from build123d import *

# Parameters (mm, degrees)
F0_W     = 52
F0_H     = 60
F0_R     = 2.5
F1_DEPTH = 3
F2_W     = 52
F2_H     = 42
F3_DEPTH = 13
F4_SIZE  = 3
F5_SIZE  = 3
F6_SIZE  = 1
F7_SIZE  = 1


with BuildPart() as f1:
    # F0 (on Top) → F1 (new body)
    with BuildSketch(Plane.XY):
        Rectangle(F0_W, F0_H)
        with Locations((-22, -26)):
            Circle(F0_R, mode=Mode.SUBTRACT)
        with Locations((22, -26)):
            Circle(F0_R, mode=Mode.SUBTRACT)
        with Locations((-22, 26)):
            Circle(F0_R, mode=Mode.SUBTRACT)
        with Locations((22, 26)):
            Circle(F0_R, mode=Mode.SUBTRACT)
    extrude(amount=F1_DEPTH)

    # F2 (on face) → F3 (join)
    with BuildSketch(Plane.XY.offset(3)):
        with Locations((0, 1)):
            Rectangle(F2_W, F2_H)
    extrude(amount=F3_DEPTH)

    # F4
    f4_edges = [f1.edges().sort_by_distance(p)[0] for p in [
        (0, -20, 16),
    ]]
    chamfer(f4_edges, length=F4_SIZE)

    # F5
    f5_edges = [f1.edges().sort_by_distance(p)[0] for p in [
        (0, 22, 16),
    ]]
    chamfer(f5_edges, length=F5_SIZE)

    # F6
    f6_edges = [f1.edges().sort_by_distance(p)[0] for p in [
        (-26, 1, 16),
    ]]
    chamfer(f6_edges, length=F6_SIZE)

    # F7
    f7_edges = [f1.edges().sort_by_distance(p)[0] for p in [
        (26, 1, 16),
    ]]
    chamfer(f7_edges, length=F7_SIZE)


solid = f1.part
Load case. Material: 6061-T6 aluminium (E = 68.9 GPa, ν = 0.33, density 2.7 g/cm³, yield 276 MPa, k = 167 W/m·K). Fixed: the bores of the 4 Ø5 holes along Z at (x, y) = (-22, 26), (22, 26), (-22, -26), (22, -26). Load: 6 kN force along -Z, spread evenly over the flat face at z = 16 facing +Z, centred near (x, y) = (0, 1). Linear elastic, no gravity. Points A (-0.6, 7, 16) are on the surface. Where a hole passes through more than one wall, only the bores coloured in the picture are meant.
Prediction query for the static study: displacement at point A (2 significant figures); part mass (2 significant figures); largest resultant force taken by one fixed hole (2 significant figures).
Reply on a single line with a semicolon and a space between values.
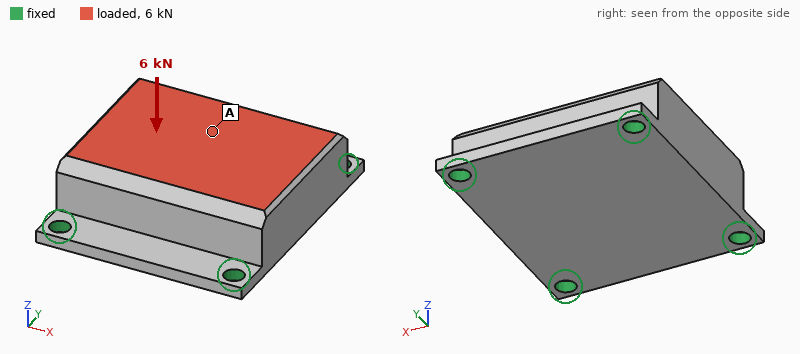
26 µm; 100 g; 1.9 kN
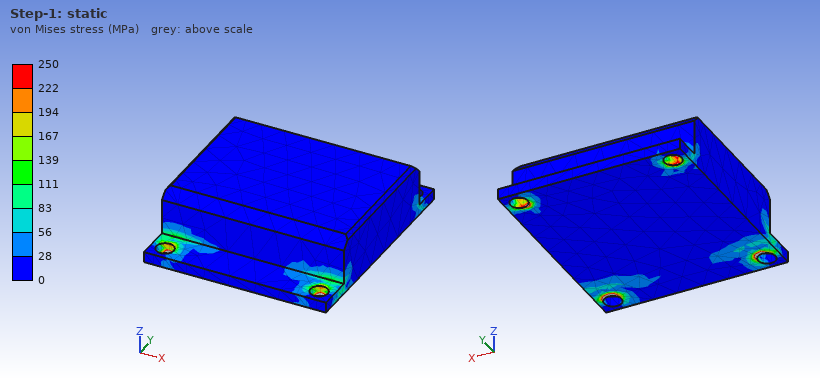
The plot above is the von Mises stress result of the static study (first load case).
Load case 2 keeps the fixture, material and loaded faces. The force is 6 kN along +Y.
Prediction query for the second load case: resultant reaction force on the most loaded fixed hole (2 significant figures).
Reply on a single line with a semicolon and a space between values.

1.9 kN
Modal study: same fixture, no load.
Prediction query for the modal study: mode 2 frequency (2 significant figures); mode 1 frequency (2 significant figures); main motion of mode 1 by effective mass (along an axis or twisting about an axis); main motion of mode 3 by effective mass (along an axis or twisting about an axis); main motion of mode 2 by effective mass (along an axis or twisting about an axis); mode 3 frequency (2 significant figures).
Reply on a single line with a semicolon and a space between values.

10 kHz; 7900 Hz; along Z; along Y; along X; 13 kHz
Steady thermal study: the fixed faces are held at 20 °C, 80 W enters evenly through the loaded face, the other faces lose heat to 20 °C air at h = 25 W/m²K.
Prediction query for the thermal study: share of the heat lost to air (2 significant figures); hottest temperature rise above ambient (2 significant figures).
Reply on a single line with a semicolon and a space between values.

3.8 %; 24 K
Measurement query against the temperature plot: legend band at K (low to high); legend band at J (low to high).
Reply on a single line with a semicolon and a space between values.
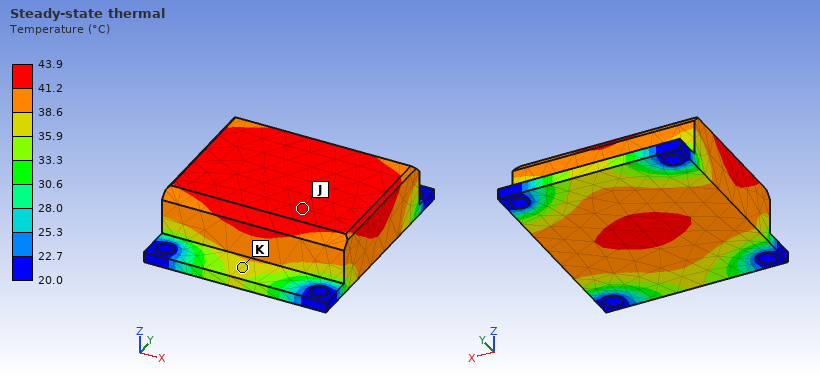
35.9 to 38.6 °C; 41.2 to 43.9 °C
